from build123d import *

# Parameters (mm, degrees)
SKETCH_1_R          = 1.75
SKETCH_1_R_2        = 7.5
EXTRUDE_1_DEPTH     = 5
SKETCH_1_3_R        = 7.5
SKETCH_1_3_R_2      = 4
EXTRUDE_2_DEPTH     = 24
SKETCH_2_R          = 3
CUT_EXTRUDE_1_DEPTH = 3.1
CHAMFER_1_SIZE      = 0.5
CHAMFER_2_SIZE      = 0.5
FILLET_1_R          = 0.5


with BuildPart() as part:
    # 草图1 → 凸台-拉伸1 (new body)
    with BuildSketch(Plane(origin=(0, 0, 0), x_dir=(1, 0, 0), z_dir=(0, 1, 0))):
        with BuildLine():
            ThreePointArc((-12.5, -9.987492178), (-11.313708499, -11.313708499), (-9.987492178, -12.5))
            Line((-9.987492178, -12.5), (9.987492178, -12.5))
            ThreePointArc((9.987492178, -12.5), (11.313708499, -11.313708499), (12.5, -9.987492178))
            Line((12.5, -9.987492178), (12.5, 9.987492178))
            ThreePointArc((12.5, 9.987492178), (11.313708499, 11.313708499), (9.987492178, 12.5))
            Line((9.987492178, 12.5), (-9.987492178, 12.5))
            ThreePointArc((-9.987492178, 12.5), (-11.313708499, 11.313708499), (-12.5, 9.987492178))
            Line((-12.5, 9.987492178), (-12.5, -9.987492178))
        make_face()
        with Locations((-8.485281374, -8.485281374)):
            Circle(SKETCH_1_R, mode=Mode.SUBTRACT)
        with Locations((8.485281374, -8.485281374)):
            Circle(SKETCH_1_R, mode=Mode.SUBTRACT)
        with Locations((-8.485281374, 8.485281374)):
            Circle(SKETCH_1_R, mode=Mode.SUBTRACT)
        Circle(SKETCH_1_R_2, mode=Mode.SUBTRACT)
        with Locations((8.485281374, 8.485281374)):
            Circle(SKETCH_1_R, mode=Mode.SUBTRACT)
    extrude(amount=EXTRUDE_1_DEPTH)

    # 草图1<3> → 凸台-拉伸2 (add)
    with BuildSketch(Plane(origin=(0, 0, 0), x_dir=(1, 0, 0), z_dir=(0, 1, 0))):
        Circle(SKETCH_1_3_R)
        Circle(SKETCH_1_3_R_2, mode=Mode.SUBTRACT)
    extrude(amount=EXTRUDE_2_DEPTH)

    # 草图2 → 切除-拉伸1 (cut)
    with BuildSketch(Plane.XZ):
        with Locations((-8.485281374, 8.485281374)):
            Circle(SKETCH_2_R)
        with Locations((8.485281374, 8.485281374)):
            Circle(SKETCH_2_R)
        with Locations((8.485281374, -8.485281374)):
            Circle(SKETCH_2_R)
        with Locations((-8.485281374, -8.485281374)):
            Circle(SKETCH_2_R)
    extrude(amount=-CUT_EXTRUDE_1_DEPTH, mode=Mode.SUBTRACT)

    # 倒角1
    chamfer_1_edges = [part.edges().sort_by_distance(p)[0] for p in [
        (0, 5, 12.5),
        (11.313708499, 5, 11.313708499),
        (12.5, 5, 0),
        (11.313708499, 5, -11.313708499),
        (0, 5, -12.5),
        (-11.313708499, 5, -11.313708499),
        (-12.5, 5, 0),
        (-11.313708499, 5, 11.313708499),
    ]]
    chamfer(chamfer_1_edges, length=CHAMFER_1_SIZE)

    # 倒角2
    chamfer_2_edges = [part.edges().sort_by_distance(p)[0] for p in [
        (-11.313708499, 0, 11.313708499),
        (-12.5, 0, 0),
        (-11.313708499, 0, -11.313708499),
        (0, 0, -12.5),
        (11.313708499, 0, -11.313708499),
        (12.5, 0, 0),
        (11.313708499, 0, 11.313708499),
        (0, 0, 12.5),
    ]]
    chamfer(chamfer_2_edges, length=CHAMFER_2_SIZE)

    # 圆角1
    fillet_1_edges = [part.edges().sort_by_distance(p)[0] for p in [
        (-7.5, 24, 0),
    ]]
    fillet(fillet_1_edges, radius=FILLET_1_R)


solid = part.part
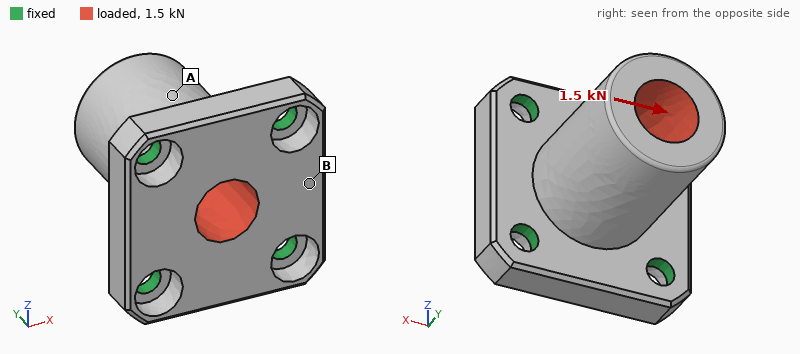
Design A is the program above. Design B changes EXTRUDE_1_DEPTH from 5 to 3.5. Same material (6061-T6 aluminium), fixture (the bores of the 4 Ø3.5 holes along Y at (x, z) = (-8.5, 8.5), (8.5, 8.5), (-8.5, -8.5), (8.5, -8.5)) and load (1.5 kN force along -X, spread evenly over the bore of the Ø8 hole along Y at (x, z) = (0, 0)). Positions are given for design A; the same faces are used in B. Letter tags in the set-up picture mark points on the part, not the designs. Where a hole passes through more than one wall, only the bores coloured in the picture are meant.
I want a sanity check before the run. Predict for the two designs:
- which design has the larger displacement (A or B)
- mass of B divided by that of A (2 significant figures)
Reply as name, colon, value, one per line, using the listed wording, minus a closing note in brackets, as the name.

which design has the larger displacement: B
mass of B divided by that of A: 0.87
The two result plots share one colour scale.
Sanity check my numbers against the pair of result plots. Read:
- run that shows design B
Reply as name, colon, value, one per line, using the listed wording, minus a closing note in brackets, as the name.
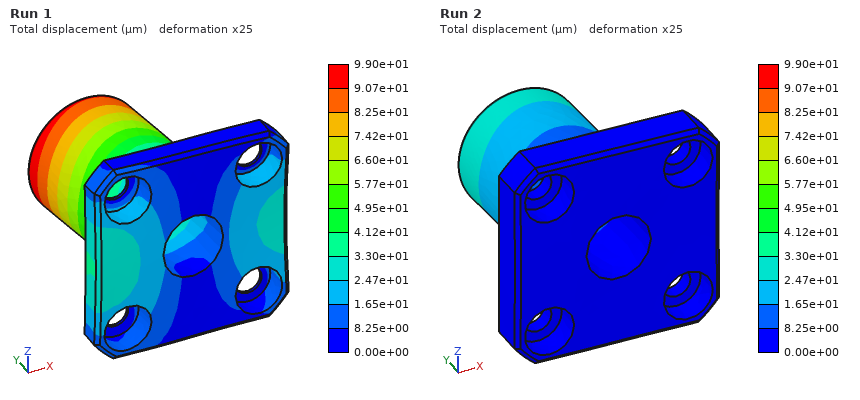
run that shows design B: Run 1
